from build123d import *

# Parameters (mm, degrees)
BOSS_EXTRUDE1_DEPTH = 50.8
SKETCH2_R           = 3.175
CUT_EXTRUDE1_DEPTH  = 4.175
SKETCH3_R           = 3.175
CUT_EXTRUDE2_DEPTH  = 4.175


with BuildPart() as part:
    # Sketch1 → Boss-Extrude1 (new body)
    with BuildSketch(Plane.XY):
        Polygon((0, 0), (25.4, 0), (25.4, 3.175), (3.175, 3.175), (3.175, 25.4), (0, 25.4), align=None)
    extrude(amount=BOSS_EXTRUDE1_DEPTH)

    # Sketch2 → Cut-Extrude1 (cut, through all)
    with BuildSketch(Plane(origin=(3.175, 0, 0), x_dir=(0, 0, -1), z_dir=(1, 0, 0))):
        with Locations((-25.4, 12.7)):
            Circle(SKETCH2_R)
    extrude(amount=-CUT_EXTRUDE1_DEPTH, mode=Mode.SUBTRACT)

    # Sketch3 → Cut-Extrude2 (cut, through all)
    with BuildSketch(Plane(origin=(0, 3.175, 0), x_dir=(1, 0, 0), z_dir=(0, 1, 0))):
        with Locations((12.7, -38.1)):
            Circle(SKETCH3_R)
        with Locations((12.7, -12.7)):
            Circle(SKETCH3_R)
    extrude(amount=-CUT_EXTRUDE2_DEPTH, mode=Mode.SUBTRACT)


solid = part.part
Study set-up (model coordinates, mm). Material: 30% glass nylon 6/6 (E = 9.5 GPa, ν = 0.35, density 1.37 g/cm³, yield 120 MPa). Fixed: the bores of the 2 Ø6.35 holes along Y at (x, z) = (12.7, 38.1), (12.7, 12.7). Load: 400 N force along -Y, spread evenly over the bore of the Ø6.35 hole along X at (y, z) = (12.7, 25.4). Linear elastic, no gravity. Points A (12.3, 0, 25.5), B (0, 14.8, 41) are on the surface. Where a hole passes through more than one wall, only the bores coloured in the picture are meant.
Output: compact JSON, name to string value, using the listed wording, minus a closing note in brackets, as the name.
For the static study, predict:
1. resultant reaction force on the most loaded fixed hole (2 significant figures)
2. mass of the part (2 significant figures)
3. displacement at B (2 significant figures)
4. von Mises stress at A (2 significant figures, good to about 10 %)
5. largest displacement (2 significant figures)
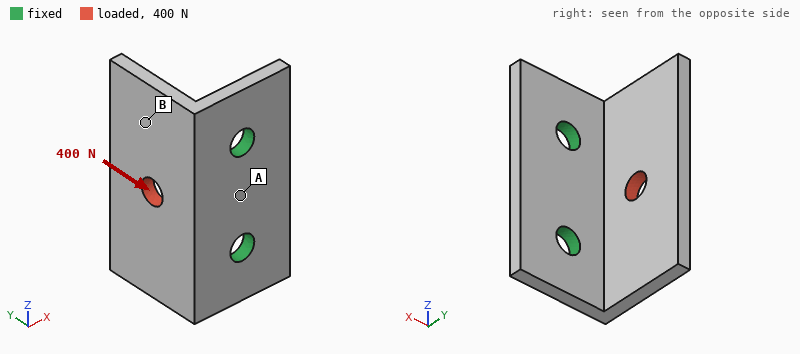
{"resultant reaction force on the most loaded fixed hole": "200 N", "mass of the part": "10 g", "displacement at B": "0.23 mm", "von Mises stress at A": "12 MPa", "largest displacement": "0.38 mm"}
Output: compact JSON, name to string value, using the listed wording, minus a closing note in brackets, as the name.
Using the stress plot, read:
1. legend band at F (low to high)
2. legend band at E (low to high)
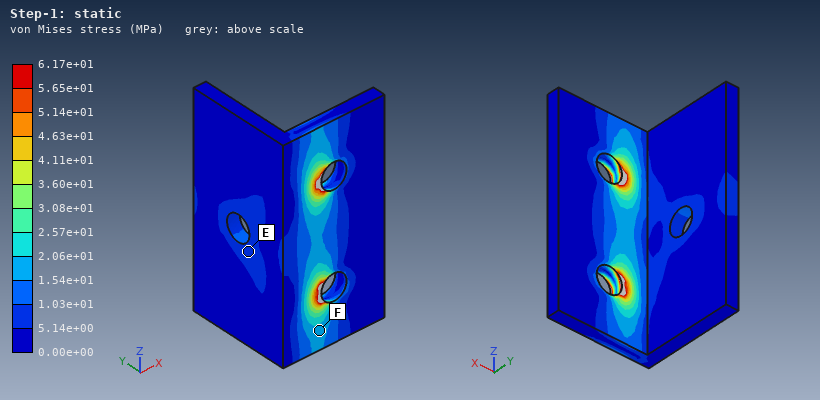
{"legend band at F": "1.54e+01 to 2.06e+01 MPa", "legend band at E": "5.14e+00 to 1.03e+01 MPa"}
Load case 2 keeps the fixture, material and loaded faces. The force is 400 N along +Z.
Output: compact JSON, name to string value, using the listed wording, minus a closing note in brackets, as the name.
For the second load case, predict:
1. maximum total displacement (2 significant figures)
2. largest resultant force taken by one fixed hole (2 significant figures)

{"maximum total displacement": "0.19 mm", "largest resultant force taken by one fixed hole": "280 N"}
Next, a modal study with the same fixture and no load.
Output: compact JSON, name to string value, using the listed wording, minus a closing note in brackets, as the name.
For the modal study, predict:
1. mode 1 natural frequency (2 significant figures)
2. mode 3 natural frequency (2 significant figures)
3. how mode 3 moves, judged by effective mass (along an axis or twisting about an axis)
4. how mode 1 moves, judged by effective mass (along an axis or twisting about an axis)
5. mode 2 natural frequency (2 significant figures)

{"mode 1 natural frequency": "1500 Hz", "mode 3 natural frequency": "4200 Hz", "how mode 3 moves, judged by effective mass": "along Z", "how mode 1 moves, judged by effective mass": "along X", "mode 2 natural frequency": "2500 Hz"}
